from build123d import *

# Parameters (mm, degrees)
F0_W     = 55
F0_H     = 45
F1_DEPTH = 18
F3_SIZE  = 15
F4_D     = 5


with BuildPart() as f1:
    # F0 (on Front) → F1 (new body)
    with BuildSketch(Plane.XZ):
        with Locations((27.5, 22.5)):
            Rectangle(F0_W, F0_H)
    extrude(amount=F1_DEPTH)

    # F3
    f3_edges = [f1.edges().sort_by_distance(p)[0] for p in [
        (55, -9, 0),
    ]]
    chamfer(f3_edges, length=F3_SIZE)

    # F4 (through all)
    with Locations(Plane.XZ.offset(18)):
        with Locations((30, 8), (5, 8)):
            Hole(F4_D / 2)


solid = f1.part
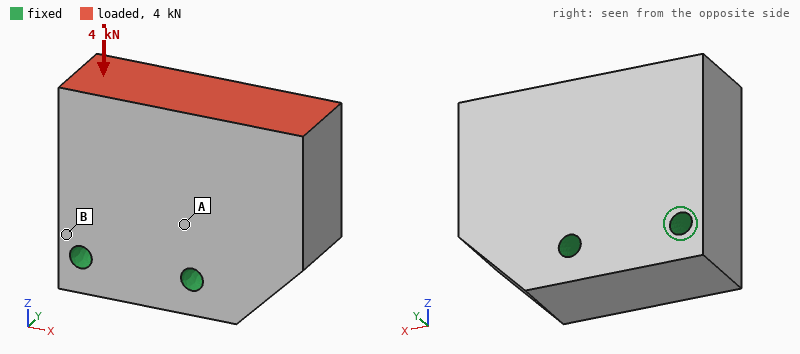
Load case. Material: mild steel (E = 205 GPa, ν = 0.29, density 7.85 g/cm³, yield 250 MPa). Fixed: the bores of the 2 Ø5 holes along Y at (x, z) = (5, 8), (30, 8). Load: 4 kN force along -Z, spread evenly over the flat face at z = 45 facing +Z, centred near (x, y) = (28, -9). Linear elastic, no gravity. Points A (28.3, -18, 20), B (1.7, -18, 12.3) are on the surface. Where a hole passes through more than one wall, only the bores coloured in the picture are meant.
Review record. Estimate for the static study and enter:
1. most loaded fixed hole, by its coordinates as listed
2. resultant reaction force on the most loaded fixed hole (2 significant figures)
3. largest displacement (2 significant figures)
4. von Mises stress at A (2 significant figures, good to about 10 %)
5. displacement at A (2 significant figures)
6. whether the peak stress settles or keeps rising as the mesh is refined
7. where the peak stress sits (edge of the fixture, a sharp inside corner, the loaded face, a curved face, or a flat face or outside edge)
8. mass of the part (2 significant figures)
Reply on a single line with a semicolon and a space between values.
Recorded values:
(30, 8); 3.4 kN; 2.6 µm; 8.0 MPa; 0.61 µm; keeps rising; edge of the fixture; 330 g
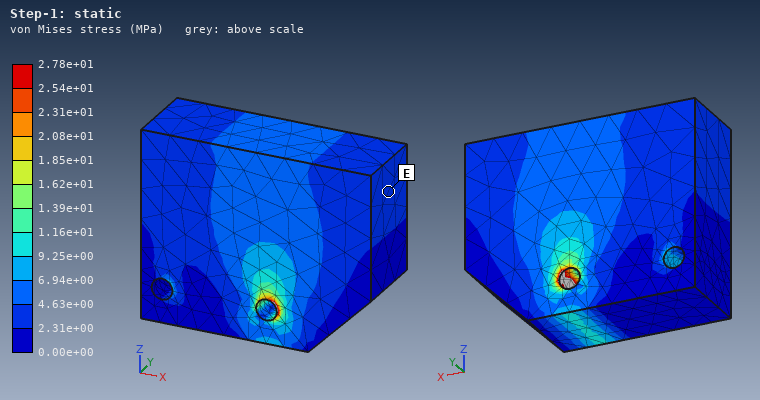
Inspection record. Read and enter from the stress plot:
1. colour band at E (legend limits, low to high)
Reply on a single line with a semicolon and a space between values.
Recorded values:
2.31e+00 to 4.63e+00 MPa
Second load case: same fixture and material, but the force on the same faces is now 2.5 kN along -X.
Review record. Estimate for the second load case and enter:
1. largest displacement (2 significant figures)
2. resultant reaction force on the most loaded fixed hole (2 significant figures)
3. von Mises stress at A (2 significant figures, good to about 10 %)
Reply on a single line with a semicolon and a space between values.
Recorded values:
5.9 µm; 3.5 kN; 9.9 MPa
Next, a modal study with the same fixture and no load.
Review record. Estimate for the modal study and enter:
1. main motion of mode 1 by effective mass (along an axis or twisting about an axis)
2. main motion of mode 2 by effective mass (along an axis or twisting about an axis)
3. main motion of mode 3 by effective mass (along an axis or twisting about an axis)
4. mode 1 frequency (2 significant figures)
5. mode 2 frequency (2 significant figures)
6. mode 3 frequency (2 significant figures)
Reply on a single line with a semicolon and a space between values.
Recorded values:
along Y; along X; twisting about Z; 7300 Hz; 11 kHz; 12 kHz
